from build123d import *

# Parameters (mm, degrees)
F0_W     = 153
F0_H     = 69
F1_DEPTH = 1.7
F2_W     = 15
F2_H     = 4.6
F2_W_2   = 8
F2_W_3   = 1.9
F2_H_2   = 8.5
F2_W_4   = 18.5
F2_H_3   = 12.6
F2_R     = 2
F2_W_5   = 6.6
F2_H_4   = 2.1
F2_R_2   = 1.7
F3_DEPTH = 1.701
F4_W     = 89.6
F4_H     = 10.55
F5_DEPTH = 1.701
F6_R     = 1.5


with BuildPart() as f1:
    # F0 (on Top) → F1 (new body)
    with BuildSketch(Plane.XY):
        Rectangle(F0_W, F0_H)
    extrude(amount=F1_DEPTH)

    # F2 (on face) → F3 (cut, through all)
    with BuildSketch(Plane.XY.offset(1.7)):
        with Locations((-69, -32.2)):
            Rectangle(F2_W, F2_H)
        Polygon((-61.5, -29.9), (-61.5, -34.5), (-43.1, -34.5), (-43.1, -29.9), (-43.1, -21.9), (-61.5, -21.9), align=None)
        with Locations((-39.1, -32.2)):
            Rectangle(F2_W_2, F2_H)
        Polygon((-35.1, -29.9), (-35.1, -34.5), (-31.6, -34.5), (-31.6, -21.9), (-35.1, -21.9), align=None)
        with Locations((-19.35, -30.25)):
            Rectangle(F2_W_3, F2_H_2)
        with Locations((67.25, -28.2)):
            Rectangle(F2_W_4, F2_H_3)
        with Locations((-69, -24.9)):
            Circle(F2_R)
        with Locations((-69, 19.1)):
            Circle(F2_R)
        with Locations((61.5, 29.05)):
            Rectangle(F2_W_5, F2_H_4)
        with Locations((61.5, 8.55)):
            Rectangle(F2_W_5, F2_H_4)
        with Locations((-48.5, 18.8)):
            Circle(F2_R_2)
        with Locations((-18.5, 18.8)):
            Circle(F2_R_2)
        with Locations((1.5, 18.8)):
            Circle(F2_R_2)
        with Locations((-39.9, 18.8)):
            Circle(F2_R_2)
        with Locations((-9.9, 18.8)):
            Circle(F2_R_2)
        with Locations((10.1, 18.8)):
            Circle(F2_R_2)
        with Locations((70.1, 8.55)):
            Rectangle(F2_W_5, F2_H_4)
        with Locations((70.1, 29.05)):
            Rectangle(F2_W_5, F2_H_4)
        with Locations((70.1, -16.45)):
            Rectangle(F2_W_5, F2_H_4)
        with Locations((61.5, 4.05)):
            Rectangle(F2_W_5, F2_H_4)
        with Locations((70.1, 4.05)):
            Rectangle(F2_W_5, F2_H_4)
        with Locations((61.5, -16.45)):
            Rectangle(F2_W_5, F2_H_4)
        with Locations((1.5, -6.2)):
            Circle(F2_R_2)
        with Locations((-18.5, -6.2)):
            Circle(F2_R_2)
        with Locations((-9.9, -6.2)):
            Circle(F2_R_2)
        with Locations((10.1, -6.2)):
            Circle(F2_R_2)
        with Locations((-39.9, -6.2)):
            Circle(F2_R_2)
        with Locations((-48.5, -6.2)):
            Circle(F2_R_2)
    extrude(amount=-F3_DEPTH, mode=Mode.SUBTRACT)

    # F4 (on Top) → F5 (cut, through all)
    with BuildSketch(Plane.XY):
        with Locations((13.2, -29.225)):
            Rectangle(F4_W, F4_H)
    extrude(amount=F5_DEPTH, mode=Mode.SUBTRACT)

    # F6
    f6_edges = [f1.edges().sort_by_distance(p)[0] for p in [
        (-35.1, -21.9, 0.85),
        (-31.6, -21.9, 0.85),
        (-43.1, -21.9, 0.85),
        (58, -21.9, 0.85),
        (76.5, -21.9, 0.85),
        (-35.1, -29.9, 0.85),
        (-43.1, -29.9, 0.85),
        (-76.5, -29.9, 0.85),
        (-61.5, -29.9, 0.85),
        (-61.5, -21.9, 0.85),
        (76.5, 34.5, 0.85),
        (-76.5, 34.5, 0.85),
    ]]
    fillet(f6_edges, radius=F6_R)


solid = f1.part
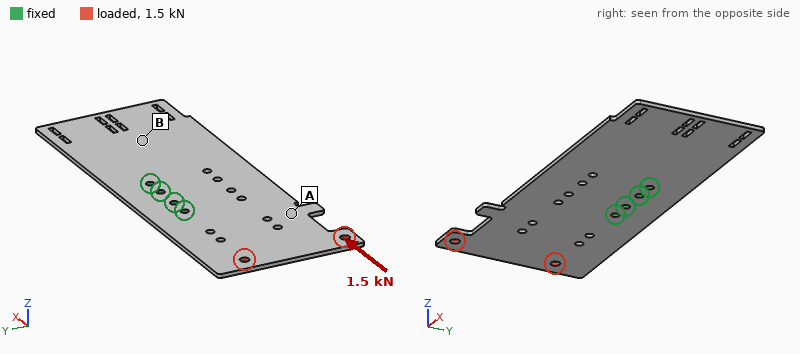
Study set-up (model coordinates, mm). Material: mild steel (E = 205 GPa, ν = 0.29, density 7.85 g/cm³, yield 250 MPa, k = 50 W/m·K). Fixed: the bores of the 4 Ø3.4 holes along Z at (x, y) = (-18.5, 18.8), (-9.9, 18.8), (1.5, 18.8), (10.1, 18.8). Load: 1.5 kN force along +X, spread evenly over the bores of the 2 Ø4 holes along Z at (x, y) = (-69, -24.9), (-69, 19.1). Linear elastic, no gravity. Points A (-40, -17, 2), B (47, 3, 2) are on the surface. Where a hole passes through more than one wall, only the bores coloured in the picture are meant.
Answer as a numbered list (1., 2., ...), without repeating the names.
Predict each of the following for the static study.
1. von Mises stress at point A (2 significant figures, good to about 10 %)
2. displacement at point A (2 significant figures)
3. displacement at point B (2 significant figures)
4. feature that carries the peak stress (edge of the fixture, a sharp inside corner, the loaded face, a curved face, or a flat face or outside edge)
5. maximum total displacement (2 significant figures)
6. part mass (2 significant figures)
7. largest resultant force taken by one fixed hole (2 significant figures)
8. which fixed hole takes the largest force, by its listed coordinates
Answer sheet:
1. 33 MPa
2. 18 µm
3. 12 µm
4. a curved face
5. 44 µm
6. 120 g
7. 1.2 kN
8. (-18.5, 18.8)
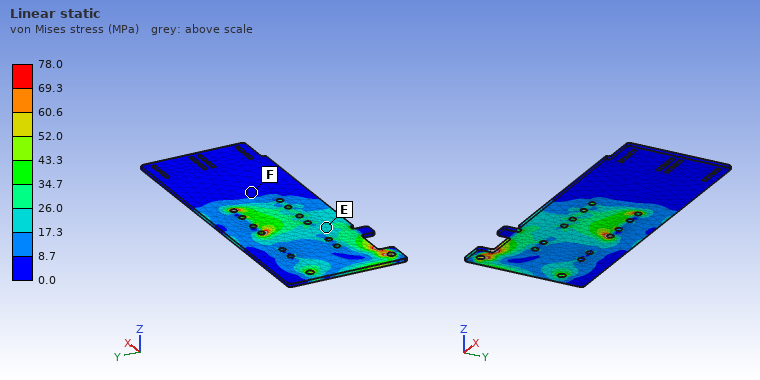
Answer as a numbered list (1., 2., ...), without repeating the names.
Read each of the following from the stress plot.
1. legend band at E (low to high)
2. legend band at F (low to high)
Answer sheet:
1. 17.3 to 26.0 MPa
2. 0.0 to 8.7 MPa
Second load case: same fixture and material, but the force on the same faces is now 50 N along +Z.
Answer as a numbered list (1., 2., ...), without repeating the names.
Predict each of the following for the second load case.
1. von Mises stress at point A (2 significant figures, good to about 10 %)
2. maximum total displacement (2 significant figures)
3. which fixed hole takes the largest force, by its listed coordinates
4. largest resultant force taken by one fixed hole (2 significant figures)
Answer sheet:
1. 49 MPa
2. 0.97 mm
3. (-18.5, 18.8)
4. 150 N
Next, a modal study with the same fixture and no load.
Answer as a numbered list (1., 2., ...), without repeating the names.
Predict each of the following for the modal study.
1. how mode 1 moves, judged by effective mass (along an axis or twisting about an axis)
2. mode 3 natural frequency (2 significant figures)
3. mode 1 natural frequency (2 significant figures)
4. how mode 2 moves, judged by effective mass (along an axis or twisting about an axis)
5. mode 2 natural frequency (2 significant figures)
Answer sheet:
1. along Z
2. 570 Hz
3. 290 Hz
4. along Z
5. 330 Hz
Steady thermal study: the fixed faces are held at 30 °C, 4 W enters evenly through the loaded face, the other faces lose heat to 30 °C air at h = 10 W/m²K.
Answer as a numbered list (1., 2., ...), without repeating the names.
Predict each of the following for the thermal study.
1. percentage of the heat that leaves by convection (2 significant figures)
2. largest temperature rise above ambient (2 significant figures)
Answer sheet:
1. 46 %
2. 54 K
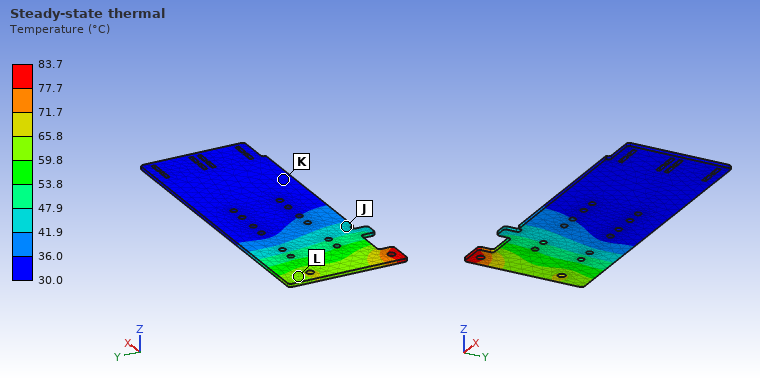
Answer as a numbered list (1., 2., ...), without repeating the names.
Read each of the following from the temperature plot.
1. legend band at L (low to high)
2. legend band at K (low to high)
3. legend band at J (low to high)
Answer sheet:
1. 59.8 to 65.8 °C
2. 30.0 to 36.0 °C
3. 41.9 to 47.9 °C
